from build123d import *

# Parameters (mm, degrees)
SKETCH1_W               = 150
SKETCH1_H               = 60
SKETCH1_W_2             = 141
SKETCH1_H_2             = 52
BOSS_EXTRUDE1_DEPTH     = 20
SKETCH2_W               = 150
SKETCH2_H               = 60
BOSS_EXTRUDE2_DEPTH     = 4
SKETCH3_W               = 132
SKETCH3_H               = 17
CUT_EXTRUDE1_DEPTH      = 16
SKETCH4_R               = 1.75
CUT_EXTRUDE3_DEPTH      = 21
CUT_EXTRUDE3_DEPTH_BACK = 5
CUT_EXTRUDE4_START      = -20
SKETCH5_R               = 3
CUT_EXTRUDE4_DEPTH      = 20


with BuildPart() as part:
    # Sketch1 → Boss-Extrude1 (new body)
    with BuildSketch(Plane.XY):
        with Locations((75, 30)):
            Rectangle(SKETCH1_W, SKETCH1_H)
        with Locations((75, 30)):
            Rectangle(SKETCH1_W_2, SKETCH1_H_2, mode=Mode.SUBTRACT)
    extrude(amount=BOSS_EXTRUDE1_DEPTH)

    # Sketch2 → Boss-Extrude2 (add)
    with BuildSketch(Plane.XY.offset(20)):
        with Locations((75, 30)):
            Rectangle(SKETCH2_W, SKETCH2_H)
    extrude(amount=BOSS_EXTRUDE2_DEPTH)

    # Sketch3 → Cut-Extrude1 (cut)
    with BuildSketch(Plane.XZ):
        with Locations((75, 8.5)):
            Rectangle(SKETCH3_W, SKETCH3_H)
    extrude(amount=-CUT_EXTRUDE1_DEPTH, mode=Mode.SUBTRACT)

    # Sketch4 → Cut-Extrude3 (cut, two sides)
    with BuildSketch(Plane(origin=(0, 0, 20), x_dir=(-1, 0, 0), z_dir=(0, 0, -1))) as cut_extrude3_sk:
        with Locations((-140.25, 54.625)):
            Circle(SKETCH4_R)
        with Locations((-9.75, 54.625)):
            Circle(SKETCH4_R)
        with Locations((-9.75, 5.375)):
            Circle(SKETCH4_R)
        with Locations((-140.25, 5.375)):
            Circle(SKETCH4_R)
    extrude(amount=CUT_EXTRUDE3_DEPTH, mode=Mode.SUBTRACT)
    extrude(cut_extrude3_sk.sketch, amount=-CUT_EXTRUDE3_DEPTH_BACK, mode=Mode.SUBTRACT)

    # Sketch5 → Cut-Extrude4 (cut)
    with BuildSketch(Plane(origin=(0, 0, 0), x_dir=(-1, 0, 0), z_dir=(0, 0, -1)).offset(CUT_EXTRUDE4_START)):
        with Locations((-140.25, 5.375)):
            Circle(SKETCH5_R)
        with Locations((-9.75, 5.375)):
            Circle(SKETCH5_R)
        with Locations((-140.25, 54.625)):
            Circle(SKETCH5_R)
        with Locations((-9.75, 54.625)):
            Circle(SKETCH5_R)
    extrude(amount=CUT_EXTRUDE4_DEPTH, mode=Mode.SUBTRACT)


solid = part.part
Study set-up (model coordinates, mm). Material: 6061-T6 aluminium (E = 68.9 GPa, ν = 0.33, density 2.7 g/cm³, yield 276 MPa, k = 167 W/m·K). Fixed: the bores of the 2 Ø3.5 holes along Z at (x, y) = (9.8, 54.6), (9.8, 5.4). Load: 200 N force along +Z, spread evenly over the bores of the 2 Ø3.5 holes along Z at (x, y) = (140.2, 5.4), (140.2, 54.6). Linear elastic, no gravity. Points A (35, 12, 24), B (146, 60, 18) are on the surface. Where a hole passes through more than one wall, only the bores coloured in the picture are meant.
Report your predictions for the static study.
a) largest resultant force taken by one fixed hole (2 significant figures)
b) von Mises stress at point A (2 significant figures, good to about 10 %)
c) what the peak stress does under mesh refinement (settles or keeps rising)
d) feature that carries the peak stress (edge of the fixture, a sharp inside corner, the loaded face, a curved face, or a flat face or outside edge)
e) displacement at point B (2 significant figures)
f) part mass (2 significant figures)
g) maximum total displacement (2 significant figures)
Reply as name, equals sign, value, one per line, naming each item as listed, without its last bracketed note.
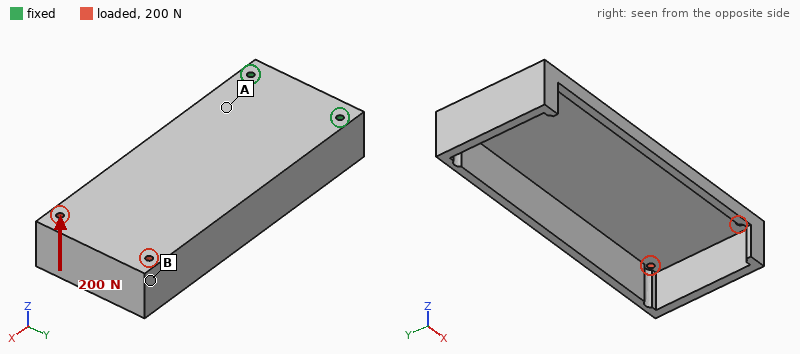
largest resultant force taken by one fixed hole = 140 N
von Mises stress at point A = 24 MPa
what the peak stress does under mesh refinement = keeps rising
feature that carries the peak stress = edge of the fixture
displacement at point B = 1.1 mm
part mass = 160 g
maximum total displacement = 1.6 mm
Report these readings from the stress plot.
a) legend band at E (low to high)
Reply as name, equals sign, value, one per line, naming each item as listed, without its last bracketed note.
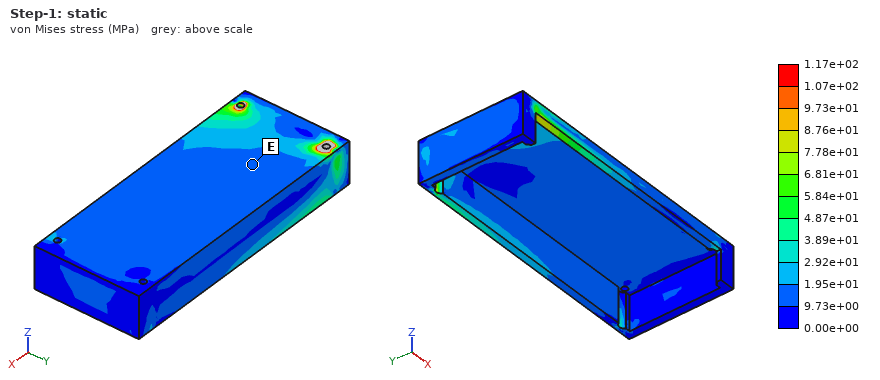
legend band at E = 9.73e+00 to 1.95e+01 MPa
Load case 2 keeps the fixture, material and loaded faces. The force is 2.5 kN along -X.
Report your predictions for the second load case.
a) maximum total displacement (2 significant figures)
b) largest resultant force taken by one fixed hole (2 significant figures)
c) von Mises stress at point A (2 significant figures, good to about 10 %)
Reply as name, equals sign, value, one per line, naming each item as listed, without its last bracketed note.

maximum total displacement = 0.12 mm
largest resultant force taken by one fixed hole = 1.3 kN
von Mises stress at point A = 12 MPa
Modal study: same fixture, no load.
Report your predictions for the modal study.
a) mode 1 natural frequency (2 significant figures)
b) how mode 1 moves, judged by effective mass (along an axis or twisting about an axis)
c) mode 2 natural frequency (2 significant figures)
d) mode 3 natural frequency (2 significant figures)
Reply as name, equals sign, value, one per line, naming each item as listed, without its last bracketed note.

mode 1 natural frequency = 260 Hz
how mode 1 moves, judged by effective mass = along Z
mode 2 natural frequency = 670 Hz
mode 3 natural frequency = 1700 Hz
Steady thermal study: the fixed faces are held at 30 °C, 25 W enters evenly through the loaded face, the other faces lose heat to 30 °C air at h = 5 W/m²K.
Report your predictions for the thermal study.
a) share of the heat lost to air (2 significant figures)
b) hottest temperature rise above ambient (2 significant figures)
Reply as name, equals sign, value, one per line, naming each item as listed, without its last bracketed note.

share of the heat lost to air = 18 %
hottest temperature rise above ambient = 62 K
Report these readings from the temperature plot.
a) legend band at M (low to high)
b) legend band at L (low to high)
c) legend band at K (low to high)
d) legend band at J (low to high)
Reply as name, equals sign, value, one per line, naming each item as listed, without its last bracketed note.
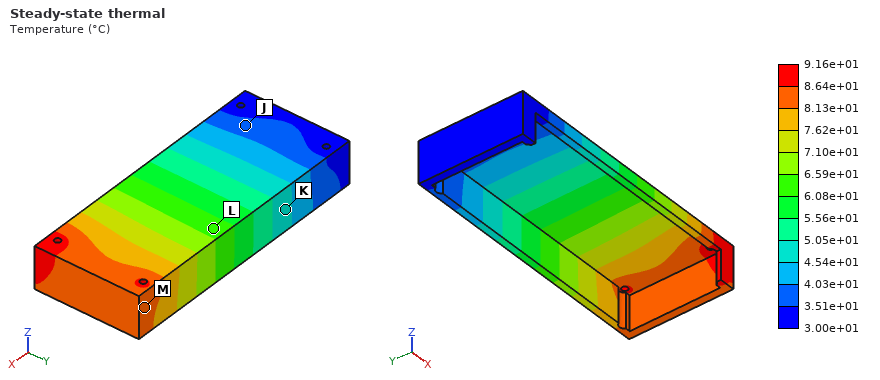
legend band at M = 8.13e+01 to 8.64e+01 °C
legend band at L = 6.08e+01 to 6.59e+01 °C
legend band at K = 4.54e+01 to 5.05e+01 °C
legend band at J = 3.51e+01 to 4.03e+01 °C
